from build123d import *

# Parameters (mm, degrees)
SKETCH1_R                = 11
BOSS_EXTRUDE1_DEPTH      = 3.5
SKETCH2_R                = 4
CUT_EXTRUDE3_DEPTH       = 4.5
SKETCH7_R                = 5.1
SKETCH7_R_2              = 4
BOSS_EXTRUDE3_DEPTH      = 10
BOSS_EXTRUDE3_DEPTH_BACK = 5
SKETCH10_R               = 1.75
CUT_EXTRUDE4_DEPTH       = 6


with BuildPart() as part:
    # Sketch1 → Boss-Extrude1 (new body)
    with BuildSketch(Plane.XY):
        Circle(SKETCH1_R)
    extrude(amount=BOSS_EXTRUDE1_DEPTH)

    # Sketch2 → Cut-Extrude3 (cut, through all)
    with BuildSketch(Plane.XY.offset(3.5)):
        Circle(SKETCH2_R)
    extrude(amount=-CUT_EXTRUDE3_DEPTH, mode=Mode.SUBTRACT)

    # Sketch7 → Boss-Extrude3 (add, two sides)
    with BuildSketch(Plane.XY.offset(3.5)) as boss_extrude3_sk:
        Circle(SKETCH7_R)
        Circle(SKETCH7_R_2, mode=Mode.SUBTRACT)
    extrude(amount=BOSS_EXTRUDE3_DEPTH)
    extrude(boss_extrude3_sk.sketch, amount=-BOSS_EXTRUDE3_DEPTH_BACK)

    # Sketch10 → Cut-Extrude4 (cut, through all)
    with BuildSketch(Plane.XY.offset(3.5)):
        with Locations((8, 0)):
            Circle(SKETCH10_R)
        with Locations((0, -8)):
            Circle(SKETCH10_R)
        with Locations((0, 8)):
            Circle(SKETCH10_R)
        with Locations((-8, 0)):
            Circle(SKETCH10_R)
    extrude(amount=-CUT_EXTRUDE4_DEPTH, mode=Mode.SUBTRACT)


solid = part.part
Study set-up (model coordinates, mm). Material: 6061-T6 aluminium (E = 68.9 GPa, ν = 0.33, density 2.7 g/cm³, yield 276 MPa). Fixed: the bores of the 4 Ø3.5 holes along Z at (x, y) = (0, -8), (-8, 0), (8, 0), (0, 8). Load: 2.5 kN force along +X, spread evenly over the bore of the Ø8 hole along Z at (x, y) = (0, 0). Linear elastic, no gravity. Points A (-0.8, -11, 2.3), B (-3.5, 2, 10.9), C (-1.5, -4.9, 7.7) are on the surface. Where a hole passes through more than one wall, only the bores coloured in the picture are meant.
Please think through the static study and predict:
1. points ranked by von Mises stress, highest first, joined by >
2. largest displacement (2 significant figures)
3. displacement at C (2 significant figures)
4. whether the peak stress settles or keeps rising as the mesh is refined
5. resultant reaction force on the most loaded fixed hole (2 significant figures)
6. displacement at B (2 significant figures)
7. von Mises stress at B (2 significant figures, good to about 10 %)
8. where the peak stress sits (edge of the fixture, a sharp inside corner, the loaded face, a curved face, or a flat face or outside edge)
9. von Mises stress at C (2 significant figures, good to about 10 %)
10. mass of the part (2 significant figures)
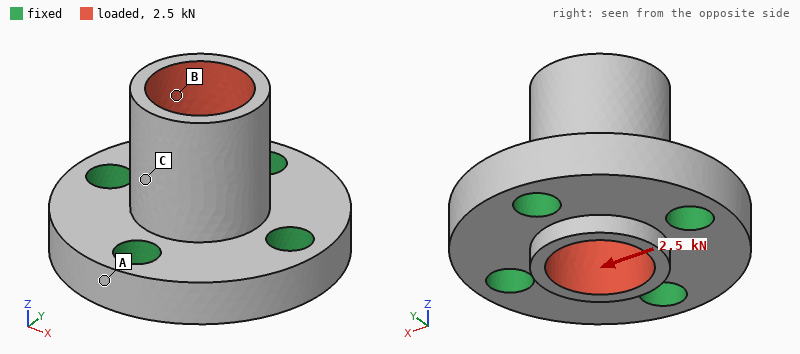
C > B > A
43 µm
21 µm
keeps rising
1.0 kN
35 µm
43 MPa
a sharp inside corner
91 MPa
3.7 g
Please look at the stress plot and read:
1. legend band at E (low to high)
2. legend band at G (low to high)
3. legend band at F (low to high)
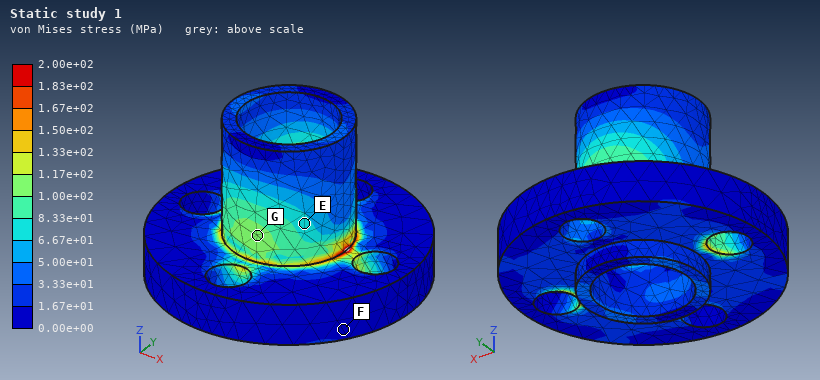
6.67e+01 to 8.33e+01 MPa
1.00e+02 to 1.17e+02 MPa
0.00e+00 to 1.67e+01 MPa
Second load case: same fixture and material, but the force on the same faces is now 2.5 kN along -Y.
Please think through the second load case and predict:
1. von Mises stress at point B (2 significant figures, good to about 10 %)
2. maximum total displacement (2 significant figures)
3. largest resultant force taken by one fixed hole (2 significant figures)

51 MPa
43 µm
1.0 kN
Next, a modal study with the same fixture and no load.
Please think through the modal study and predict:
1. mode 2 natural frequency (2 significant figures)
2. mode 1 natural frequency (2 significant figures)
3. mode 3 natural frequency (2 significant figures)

39 kHz
39 kHz
42 kHz
